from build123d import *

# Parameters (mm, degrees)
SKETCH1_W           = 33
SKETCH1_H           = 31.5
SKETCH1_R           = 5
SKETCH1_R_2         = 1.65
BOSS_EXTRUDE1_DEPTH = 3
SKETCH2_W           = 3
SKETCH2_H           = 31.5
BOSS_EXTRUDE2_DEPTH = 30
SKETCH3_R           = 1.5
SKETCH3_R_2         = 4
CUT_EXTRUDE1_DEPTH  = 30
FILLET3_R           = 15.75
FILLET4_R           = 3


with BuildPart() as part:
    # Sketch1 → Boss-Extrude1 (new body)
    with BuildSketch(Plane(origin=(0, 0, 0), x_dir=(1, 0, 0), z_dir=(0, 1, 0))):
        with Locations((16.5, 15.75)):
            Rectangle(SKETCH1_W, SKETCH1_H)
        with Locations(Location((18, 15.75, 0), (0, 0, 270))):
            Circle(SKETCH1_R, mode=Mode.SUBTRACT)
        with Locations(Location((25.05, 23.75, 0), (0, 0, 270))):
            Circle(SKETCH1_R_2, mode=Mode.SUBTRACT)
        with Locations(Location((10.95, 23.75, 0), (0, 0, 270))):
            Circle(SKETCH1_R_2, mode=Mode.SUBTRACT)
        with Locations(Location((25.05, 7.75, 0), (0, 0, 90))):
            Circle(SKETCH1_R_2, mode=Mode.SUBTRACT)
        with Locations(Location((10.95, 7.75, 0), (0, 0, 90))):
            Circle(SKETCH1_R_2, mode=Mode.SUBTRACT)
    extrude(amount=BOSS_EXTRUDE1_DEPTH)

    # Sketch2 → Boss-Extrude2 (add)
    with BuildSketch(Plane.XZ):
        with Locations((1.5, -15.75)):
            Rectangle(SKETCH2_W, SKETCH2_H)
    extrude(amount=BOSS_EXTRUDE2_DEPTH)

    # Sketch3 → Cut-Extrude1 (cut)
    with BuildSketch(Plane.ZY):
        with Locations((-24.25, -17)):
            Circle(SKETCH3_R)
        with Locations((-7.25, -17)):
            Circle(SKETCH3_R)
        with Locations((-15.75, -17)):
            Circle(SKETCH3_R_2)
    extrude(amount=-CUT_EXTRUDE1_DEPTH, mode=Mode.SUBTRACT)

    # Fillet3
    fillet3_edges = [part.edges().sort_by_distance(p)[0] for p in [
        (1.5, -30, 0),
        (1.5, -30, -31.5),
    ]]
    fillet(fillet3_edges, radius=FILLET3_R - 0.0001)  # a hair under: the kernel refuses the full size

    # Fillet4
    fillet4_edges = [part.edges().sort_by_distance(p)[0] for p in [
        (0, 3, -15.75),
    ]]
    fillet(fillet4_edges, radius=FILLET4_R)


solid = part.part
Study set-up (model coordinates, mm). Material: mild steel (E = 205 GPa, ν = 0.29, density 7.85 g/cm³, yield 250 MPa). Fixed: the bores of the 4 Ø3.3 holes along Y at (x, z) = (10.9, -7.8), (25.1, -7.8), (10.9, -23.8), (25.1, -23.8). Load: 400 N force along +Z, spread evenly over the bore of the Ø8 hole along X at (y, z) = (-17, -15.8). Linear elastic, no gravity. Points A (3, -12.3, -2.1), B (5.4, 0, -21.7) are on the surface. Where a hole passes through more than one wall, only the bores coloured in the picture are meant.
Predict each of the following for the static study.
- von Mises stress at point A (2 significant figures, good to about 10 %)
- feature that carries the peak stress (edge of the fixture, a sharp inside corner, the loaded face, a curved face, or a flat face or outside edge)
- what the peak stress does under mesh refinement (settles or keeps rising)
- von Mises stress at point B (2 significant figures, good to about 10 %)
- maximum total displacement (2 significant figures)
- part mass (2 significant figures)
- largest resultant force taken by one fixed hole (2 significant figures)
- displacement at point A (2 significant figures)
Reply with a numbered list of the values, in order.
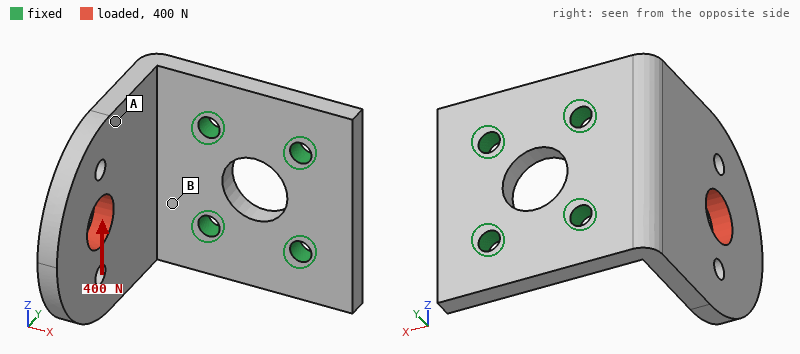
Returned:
1. 15 MPa
2. edge of the fixture
3. keeps rising
4. 55 MPa
5. 32 µm
6. 40 g
7. 470 N
8. 21 µm
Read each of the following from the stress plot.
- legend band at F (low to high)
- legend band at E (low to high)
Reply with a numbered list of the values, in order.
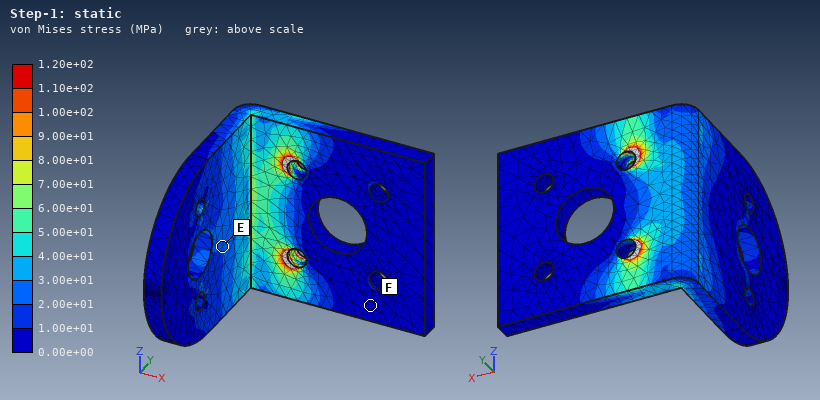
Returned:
1. 0.00e+00 to 1.00e+01 MPa
2. 2.00e+01 to 3.00e+01 MPa
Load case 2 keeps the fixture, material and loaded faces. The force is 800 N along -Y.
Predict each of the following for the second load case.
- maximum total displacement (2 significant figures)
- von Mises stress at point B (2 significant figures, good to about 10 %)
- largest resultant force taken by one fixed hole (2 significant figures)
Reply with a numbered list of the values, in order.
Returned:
1. 78 µm
2. 63 MPa
3. 450 N
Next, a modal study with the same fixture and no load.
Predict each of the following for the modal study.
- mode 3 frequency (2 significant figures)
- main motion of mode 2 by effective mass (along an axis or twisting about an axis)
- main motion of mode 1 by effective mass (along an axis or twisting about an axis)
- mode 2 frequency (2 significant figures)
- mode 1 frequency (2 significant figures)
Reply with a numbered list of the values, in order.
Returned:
1. 7600 Hz
2. along Z
3. along X
4. 5000 Hz
5. 2100 Hz
